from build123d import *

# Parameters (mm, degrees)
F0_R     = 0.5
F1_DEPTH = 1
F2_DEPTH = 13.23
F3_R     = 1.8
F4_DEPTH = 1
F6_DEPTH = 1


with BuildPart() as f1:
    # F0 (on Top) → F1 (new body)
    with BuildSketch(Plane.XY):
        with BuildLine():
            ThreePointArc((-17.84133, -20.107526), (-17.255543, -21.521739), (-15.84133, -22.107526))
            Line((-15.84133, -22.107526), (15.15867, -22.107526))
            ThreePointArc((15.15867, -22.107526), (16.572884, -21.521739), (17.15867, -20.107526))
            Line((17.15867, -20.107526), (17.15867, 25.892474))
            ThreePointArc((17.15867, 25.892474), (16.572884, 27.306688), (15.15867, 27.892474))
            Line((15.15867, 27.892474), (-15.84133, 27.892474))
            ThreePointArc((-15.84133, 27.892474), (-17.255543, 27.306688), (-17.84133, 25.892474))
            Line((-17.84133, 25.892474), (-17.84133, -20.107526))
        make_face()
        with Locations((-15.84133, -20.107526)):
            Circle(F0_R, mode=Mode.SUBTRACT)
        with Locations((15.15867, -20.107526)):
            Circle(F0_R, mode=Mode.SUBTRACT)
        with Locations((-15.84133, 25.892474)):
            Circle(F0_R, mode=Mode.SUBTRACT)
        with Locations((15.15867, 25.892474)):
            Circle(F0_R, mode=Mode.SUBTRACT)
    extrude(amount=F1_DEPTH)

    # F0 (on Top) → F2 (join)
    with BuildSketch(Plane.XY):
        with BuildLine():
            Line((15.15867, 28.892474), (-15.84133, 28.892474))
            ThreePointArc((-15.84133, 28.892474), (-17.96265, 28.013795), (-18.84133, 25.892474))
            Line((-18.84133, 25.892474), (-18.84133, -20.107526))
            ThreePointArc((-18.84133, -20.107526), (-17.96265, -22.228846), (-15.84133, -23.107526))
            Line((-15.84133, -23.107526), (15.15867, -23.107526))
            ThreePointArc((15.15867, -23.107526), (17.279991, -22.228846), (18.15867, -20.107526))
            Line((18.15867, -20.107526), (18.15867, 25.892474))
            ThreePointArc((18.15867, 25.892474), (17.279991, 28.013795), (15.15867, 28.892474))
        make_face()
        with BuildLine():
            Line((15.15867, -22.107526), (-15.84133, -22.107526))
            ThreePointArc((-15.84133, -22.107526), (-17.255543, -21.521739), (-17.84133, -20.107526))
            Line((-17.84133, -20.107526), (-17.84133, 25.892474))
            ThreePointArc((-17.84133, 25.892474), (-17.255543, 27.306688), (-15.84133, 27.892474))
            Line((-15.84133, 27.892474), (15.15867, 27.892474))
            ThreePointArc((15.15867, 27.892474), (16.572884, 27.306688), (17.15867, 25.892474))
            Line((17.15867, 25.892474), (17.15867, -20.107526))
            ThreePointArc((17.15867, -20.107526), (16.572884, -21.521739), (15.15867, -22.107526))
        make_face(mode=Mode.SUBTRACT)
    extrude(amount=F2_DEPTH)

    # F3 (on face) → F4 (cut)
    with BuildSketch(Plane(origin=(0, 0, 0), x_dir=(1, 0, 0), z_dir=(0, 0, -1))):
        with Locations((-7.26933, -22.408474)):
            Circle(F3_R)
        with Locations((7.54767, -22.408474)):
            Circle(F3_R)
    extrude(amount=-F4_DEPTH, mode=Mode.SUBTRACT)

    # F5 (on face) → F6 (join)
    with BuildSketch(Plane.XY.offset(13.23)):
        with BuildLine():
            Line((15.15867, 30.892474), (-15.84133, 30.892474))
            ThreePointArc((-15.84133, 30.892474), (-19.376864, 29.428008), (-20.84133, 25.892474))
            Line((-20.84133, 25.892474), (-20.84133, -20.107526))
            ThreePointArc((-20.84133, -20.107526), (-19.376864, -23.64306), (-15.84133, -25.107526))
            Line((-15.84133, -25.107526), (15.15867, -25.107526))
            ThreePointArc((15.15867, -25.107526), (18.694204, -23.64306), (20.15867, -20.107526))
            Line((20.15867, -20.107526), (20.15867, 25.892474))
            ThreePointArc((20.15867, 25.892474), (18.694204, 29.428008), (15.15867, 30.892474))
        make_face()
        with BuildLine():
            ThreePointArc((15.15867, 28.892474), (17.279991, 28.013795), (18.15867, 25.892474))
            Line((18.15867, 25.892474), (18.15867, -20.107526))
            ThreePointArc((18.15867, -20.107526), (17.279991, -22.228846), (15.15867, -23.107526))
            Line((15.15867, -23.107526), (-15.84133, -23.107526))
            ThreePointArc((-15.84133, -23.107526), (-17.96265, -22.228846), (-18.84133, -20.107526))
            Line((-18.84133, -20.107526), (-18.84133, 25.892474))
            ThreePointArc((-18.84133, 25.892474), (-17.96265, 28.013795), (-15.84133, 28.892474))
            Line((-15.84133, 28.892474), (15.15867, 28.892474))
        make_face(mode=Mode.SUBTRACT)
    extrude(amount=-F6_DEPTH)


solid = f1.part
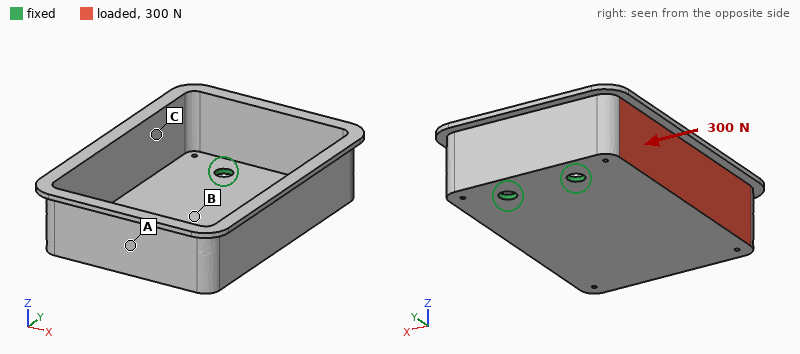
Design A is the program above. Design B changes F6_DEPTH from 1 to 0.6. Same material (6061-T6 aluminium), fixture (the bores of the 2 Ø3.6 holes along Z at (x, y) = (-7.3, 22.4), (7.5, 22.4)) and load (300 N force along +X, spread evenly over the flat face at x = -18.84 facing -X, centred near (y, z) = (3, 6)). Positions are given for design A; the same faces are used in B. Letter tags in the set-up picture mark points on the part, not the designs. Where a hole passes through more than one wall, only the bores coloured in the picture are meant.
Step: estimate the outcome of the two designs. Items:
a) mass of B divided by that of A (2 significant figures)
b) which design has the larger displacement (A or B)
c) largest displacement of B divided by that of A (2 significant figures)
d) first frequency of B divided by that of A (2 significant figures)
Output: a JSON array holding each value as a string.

["0.97", "B", "1.2", "1.0"]
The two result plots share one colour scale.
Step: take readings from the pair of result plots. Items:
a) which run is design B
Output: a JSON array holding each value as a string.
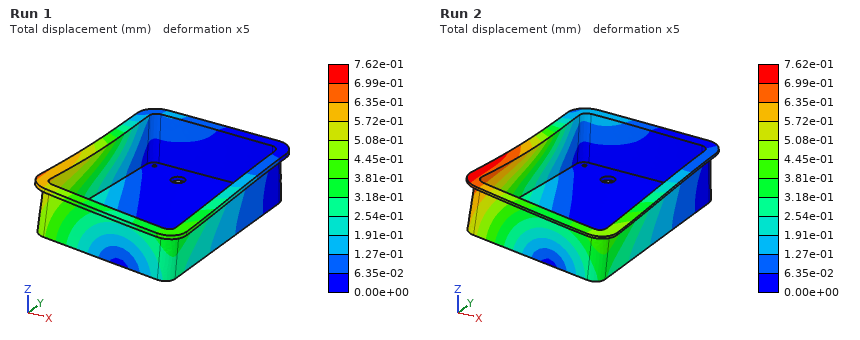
["Run 2"]
